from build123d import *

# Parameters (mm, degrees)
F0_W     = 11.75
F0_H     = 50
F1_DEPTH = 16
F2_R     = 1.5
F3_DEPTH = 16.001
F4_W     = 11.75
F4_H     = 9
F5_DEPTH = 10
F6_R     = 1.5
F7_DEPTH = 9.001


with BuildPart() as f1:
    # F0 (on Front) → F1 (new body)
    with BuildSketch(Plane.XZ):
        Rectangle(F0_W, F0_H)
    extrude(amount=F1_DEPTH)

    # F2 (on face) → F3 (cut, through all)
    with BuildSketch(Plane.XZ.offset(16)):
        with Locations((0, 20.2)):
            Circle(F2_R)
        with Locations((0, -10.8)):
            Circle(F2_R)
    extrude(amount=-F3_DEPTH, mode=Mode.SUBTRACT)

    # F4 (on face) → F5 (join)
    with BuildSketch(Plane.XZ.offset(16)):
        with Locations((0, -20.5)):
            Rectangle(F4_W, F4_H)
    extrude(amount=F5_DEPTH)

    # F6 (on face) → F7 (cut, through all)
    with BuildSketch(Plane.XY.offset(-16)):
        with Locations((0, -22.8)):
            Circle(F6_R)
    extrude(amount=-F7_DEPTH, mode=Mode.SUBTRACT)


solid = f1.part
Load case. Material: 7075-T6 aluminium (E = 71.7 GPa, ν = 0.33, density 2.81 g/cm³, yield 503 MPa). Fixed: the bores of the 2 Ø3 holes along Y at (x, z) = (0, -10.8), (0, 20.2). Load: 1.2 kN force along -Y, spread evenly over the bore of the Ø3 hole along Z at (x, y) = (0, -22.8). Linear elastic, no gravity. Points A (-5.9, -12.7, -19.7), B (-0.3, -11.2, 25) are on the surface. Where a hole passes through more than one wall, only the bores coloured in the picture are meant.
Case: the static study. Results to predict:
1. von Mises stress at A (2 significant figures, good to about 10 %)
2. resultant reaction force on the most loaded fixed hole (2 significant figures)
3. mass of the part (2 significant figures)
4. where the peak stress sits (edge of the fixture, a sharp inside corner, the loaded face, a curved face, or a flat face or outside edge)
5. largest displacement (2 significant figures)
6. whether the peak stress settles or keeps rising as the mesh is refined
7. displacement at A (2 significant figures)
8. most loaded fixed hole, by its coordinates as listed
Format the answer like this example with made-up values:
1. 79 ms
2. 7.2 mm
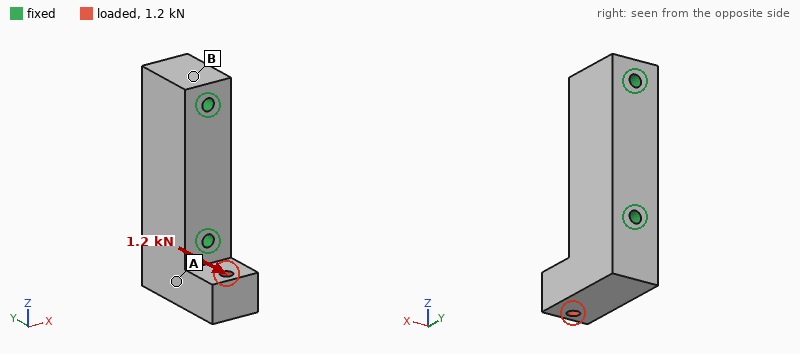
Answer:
1. 13 MPa
2. 1.2 kN
3. 29 g
4. edge of the fixture
5. 11 µm
6. keeps rising
7. 4.1 µm
8. (0, -10.8)
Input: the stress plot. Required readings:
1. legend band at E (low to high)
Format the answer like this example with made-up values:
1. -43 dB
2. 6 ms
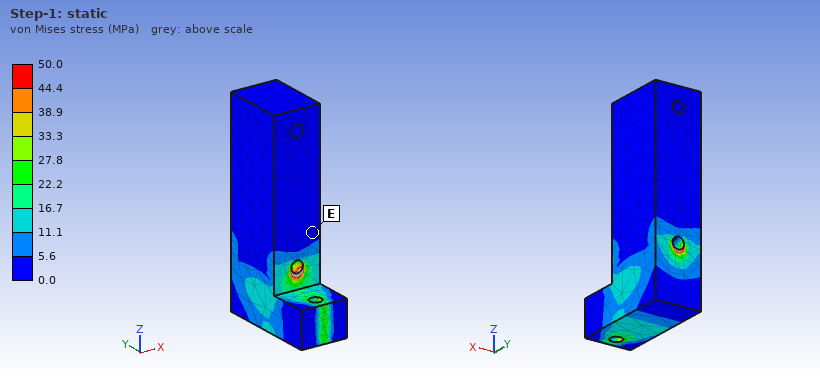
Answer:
1. 0.0 to 5.6 MPa
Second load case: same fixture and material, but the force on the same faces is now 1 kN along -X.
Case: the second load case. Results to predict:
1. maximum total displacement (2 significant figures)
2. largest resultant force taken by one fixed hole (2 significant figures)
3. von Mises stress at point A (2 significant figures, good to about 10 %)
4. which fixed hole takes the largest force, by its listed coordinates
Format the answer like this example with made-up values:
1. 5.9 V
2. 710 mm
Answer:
1. 38 µm
2. 1.2 kN
3. 38 MPa
4. (0, -10.8)
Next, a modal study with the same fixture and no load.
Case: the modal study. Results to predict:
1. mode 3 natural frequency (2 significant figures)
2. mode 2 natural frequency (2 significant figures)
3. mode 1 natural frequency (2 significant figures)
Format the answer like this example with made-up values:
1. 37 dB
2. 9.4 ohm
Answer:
1. 26 kHz
2. 22 kHz
3. 17 kHz
